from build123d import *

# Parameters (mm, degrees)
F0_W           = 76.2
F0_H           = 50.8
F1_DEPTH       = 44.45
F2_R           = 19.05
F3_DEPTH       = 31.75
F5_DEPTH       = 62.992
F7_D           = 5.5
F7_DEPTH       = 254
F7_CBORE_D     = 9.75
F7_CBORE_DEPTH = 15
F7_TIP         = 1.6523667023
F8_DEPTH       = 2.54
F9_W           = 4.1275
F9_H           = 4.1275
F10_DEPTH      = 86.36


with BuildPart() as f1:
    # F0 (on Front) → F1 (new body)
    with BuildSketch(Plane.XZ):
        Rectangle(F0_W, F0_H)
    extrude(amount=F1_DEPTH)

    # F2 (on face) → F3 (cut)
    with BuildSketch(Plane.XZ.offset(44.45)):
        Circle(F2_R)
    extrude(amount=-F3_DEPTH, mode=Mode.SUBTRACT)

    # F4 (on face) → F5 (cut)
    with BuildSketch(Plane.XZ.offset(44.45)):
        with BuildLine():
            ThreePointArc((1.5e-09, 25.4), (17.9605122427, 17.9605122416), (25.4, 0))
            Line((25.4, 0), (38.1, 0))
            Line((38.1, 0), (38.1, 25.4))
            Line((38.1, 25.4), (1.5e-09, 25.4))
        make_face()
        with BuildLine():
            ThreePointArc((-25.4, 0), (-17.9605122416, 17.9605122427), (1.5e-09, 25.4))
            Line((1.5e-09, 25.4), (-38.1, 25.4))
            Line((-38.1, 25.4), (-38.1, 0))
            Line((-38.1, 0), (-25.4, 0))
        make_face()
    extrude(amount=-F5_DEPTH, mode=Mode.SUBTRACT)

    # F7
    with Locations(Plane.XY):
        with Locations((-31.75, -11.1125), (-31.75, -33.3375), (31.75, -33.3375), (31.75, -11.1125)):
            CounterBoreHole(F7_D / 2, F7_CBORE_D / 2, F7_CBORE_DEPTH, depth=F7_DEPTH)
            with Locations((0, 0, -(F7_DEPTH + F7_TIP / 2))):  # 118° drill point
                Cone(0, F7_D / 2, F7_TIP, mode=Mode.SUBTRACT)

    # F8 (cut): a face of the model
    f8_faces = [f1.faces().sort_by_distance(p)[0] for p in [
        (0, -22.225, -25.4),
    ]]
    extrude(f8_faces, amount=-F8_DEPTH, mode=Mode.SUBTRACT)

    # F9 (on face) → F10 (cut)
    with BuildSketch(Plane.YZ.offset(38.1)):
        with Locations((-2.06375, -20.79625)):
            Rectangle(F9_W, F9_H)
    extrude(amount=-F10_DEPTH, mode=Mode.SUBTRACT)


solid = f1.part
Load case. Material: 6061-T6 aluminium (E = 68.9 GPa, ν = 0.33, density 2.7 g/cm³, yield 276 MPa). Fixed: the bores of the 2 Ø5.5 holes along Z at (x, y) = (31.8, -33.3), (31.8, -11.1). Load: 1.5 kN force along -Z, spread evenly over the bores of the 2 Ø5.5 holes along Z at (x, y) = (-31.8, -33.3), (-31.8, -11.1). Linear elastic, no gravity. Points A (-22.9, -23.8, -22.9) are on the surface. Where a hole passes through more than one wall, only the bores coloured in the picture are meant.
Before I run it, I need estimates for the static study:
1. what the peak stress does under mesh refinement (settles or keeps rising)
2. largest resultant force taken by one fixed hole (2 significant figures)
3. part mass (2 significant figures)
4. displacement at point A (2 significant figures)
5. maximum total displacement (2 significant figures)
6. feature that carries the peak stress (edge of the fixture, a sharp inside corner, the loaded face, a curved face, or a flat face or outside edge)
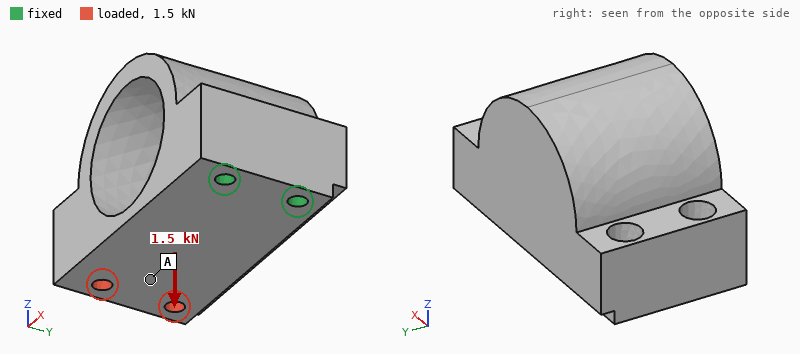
keeps rising
800 N
220 g
0.21 mm
0.28 mm
edge of the fixture
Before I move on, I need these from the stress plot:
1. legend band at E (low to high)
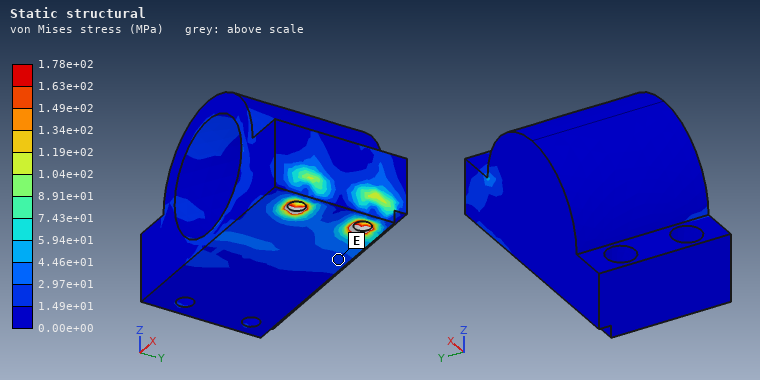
1.49e+01 to 2.97e+01 MPa
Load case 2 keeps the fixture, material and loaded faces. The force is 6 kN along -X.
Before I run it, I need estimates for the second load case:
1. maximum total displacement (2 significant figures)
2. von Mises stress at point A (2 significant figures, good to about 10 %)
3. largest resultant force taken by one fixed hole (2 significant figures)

36 µm
18 MPa
3.0 kN
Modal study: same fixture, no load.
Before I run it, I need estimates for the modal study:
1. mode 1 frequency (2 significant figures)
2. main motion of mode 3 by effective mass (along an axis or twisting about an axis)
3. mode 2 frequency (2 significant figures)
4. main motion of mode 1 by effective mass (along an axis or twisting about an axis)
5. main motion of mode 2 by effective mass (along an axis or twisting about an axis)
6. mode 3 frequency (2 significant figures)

1300 Hz
twisting about X
3000 Hz
along Z
along Y
5100 Hz
